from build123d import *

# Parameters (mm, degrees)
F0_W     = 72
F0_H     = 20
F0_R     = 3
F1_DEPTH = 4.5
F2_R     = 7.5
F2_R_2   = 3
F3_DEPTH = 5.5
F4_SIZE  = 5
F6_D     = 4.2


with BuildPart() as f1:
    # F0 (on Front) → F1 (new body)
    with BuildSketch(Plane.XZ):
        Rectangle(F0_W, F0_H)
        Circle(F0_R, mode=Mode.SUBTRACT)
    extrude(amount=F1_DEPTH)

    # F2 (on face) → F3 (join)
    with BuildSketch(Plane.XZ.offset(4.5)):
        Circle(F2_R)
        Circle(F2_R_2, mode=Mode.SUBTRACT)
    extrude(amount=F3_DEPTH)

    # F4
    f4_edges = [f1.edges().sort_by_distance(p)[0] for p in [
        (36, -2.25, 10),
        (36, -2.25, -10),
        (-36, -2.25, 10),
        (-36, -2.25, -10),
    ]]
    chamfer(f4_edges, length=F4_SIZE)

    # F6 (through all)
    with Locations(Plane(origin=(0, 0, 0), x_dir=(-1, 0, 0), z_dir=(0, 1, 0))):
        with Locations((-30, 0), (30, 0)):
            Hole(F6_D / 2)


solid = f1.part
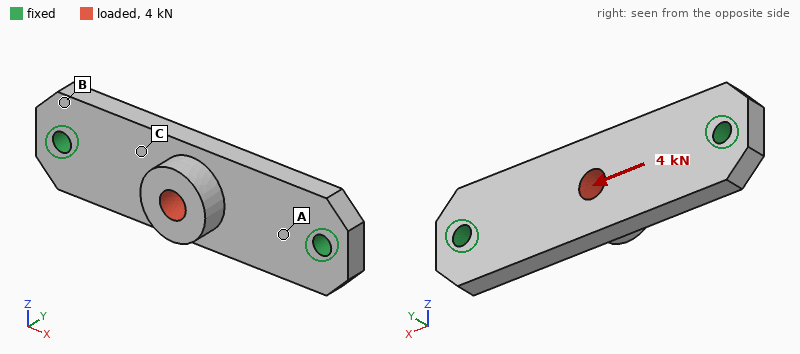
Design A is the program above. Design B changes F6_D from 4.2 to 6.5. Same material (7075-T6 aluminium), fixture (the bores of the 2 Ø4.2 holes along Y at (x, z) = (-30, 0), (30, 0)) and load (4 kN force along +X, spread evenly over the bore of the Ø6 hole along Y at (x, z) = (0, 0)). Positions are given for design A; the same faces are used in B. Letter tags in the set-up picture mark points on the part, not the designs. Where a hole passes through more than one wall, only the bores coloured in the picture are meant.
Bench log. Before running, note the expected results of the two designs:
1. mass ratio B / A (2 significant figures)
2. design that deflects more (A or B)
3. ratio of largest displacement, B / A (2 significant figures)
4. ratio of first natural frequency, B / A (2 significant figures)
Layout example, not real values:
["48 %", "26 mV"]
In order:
["0.97", "A", "0.91", "1.1"]
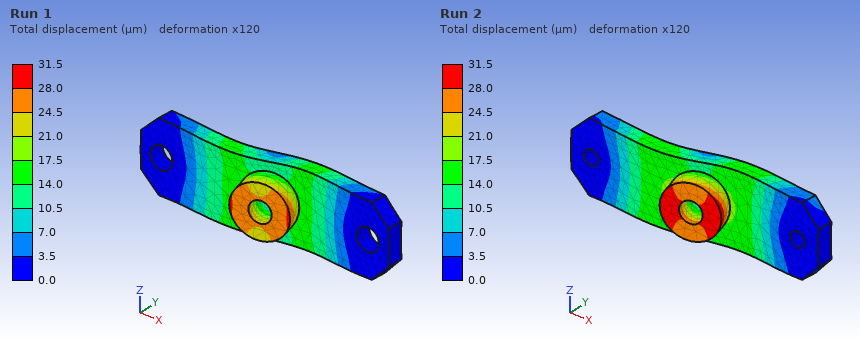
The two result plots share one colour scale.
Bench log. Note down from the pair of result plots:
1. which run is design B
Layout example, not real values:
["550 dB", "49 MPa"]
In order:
["Run 1"]
